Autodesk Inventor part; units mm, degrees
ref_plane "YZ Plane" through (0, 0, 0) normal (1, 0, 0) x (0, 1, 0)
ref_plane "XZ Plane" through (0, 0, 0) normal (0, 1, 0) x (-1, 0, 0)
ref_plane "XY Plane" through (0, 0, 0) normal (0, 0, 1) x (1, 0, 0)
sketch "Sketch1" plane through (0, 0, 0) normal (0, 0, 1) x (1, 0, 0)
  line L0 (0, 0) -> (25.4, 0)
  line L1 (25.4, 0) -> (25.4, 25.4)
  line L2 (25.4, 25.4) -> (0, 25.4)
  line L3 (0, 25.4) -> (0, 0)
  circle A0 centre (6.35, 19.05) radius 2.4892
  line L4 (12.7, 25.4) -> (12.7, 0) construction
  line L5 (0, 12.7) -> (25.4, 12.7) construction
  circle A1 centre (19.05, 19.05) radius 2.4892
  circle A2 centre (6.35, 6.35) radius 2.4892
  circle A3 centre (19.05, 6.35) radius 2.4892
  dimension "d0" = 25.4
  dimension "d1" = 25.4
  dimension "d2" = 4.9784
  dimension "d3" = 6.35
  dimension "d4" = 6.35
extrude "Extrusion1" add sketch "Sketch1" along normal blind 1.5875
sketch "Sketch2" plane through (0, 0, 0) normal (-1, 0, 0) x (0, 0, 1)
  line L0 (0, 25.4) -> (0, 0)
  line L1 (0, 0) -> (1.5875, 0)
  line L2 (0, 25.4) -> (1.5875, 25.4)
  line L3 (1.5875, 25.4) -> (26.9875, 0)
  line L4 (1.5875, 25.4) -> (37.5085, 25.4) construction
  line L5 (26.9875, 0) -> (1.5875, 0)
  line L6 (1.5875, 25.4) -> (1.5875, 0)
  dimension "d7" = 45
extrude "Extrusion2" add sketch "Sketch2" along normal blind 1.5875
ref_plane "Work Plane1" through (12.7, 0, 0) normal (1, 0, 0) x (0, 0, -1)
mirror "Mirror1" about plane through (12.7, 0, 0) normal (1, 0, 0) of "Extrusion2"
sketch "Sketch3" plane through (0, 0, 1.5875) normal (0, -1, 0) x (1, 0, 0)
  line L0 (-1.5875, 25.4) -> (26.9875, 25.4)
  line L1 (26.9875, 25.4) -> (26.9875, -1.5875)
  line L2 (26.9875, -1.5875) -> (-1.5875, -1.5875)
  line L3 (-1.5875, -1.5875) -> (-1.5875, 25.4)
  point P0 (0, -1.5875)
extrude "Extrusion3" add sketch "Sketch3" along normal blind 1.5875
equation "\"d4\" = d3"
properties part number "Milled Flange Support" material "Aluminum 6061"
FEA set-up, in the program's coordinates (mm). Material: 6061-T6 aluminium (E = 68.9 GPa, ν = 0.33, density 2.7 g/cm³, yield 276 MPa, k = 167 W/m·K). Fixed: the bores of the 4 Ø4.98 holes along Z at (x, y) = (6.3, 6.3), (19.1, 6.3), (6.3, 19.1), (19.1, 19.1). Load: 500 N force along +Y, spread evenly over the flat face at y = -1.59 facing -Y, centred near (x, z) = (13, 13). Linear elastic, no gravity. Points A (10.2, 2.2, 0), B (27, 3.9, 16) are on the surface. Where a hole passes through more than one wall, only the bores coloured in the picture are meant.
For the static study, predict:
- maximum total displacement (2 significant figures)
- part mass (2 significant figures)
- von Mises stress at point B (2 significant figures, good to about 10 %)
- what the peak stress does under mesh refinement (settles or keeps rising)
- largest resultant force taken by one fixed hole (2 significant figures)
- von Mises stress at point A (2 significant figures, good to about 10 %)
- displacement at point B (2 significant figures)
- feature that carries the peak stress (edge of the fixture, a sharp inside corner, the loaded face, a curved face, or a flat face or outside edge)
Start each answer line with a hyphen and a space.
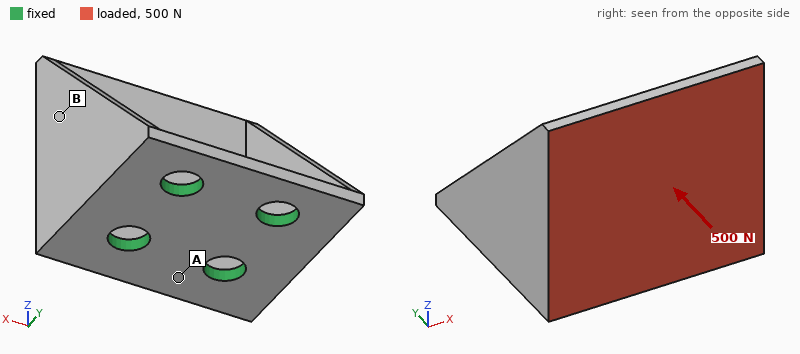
- 0.20 mm
- 8.8 g
- 27 MPa
- keeps rising
- 250 N
- 58 MPa
- 0.051 mm
- edge of the fixture
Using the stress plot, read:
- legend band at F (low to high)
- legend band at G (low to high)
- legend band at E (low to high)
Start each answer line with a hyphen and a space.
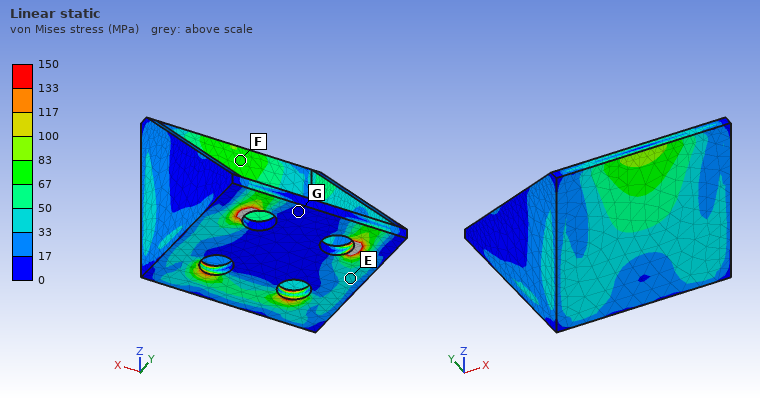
- 67 to 83 MPa
- 0 to 17 MPa
- 33 to 50 MPa
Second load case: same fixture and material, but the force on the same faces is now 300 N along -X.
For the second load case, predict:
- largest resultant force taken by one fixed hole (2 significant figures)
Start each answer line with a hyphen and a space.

- 290 N
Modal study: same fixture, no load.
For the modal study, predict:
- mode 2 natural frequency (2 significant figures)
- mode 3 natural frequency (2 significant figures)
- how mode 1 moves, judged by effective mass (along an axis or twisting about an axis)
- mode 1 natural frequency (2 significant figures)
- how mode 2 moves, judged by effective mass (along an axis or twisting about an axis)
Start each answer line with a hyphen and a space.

- 5100 Hz
- 9600 Hz
- along X
- 4900 Hz
- along Y
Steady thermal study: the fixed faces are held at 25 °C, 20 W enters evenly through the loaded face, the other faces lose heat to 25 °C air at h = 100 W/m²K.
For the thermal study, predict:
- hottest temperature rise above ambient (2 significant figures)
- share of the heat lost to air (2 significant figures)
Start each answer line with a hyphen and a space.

- 26 K
- 16 %
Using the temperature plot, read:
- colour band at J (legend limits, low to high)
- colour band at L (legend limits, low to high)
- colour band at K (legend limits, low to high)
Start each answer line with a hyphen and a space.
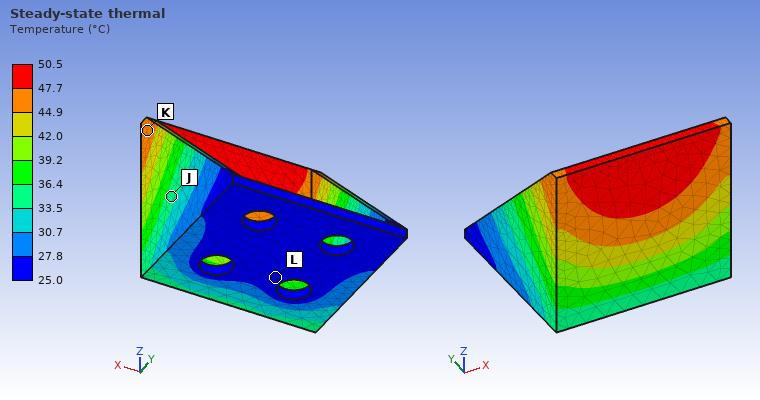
- 33.5 to 36.4 °C
- 25.0 to 27.8 °C
- 44.9 to 47.7 °C
